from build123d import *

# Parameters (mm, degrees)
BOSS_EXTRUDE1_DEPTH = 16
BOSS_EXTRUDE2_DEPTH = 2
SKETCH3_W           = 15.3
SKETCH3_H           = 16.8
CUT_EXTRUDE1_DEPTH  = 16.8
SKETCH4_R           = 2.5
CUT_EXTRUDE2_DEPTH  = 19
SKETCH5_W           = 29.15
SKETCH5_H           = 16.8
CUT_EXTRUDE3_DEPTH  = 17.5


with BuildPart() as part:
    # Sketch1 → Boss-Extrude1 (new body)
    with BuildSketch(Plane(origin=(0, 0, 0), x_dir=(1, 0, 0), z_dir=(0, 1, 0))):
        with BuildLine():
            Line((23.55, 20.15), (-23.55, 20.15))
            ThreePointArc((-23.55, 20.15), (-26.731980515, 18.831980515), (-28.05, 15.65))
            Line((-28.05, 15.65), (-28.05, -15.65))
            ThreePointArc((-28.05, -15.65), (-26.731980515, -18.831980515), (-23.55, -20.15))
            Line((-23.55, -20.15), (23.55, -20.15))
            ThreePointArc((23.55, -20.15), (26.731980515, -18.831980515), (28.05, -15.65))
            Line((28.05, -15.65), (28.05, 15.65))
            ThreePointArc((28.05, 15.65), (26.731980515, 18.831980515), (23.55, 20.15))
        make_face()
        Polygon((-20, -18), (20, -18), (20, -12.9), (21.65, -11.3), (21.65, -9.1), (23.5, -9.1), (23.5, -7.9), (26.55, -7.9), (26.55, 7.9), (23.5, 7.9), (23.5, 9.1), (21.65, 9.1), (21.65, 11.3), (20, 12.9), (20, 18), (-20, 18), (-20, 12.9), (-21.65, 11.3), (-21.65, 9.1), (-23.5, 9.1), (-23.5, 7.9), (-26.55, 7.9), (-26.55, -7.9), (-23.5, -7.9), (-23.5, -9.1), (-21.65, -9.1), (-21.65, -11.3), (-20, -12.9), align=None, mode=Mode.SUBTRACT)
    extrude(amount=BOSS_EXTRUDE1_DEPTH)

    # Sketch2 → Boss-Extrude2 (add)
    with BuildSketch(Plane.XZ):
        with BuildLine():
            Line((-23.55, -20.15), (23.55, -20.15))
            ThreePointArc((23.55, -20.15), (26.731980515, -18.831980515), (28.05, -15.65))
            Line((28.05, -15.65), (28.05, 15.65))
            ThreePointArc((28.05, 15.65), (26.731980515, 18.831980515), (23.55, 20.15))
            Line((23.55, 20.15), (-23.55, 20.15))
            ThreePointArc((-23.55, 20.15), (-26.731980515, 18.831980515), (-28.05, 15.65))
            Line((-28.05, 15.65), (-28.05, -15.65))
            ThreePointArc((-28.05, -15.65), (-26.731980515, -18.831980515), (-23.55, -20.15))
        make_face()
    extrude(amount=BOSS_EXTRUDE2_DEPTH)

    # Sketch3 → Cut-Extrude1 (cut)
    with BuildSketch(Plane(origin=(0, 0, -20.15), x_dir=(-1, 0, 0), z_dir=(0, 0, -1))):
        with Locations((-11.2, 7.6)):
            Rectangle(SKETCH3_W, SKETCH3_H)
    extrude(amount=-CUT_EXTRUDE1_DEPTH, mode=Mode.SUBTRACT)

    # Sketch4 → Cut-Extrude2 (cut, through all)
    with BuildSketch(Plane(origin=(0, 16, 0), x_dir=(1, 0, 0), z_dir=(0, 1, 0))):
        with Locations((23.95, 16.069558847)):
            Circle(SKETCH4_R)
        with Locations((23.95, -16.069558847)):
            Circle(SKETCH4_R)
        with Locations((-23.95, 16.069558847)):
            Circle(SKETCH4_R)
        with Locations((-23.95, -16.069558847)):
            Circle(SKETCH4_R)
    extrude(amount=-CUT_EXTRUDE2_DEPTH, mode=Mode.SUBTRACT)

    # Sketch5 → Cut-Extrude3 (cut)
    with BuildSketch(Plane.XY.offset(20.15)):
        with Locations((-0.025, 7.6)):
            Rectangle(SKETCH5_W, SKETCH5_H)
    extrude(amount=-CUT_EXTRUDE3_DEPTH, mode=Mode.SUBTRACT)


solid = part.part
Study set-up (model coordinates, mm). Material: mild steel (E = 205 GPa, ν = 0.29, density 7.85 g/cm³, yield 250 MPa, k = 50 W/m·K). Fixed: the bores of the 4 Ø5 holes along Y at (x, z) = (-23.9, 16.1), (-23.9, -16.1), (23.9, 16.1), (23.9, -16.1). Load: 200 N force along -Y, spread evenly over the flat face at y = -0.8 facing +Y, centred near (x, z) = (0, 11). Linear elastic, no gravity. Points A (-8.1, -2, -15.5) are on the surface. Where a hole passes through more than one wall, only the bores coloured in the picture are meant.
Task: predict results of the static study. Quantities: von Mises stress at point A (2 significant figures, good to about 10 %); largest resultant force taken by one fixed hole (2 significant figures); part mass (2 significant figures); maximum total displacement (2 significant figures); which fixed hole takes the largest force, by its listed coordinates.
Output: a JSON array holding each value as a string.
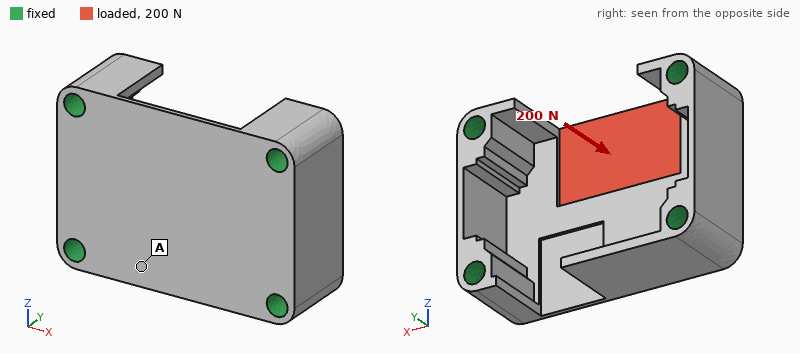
["9.3 MPa", "140 N", "78 g", "32 µm", "(23.9, 16.1)"]
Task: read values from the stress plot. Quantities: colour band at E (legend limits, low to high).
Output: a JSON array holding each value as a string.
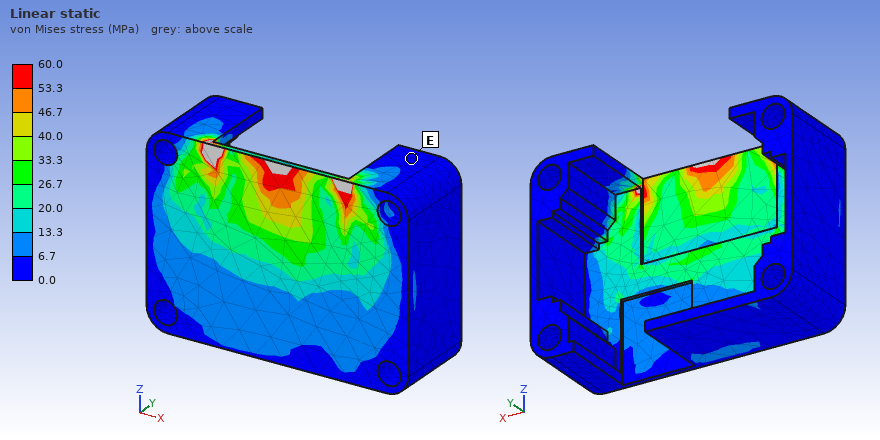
["0.0 to 6.7 MPa"]
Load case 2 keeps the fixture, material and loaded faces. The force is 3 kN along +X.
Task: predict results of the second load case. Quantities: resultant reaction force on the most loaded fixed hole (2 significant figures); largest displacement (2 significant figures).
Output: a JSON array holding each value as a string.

["1.1 kN", "6.8 µm"]
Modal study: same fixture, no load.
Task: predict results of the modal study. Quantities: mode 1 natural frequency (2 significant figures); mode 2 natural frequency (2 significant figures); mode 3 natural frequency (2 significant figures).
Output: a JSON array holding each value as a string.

["5700 Hz", "7400 Hz", "9400 Hz"]
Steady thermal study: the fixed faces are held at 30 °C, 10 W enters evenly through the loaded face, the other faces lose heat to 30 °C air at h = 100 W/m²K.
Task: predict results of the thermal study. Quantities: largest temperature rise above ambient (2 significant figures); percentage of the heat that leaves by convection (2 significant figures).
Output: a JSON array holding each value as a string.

["33 K", "33 %"]
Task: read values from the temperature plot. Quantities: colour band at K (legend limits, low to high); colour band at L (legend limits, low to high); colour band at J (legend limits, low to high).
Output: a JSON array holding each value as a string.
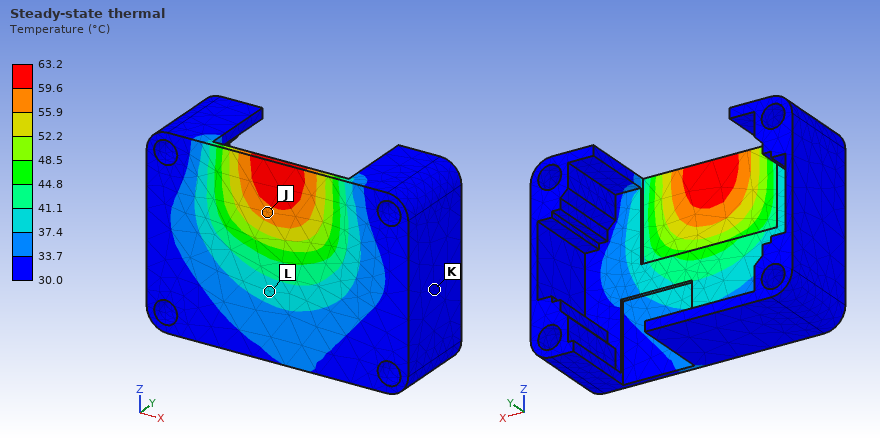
["30.0 to 33.7 °C", "37.4 to 41.1 °C", "55.9 to 59.6 °C"]
